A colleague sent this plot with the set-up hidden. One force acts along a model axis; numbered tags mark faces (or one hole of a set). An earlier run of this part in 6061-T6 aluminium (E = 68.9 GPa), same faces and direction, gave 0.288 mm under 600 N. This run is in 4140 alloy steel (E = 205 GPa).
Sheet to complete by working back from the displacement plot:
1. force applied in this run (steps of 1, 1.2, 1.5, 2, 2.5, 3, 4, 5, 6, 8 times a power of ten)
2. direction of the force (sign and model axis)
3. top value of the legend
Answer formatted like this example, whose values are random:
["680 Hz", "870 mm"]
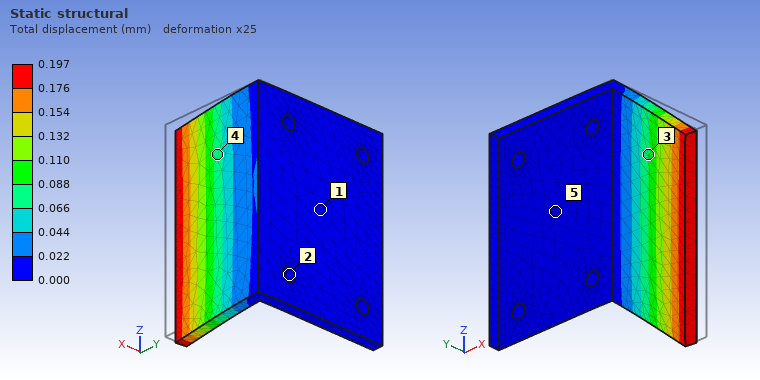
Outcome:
["1.2 kN", "-X", "0.197 mm"]
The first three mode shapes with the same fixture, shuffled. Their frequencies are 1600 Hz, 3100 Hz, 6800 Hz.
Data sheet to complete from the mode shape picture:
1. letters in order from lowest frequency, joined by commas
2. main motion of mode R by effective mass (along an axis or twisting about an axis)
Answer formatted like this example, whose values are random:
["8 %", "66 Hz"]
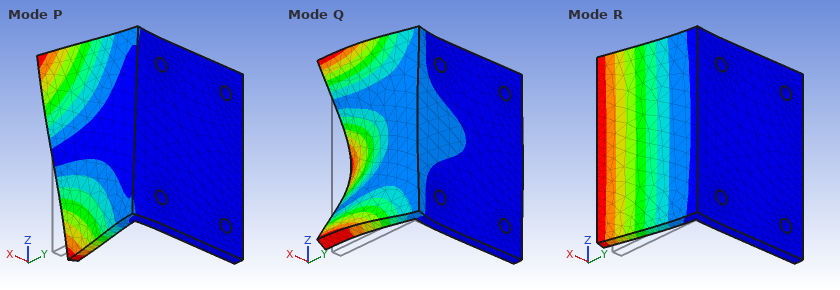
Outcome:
["R, P, Q", "along X"]
